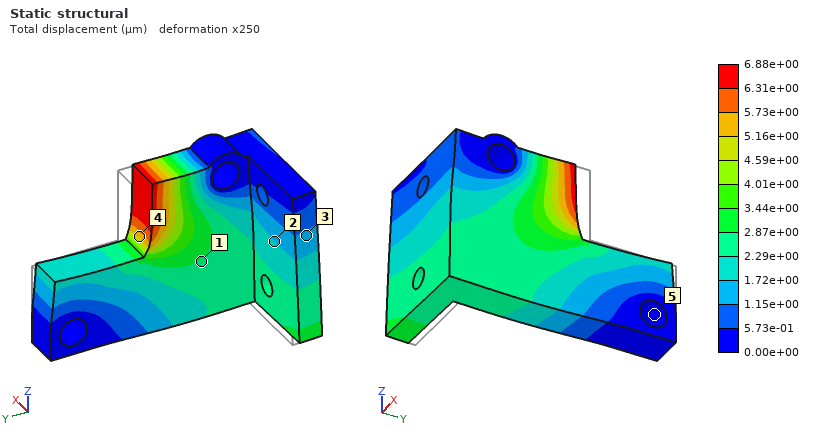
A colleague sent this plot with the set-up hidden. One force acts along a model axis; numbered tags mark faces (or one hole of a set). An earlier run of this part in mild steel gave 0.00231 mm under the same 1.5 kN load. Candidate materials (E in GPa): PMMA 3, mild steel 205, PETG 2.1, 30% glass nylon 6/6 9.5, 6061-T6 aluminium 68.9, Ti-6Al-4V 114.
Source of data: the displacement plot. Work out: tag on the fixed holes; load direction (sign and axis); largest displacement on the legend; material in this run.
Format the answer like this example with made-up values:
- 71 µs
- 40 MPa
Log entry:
- 5
- -Y
- 6.88e+00 µm
- 6061-T6 aluminium
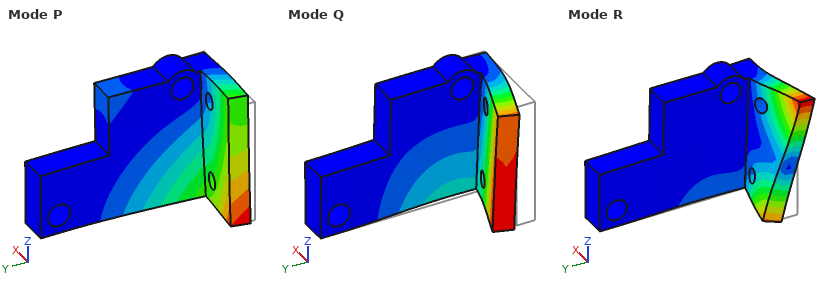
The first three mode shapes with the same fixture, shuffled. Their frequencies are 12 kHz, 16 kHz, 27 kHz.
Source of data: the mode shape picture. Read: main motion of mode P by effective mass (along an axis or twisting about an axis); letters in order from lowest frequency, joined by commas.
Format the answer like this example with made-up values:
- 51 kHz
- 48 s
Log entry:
- along X
- P, Q, R
